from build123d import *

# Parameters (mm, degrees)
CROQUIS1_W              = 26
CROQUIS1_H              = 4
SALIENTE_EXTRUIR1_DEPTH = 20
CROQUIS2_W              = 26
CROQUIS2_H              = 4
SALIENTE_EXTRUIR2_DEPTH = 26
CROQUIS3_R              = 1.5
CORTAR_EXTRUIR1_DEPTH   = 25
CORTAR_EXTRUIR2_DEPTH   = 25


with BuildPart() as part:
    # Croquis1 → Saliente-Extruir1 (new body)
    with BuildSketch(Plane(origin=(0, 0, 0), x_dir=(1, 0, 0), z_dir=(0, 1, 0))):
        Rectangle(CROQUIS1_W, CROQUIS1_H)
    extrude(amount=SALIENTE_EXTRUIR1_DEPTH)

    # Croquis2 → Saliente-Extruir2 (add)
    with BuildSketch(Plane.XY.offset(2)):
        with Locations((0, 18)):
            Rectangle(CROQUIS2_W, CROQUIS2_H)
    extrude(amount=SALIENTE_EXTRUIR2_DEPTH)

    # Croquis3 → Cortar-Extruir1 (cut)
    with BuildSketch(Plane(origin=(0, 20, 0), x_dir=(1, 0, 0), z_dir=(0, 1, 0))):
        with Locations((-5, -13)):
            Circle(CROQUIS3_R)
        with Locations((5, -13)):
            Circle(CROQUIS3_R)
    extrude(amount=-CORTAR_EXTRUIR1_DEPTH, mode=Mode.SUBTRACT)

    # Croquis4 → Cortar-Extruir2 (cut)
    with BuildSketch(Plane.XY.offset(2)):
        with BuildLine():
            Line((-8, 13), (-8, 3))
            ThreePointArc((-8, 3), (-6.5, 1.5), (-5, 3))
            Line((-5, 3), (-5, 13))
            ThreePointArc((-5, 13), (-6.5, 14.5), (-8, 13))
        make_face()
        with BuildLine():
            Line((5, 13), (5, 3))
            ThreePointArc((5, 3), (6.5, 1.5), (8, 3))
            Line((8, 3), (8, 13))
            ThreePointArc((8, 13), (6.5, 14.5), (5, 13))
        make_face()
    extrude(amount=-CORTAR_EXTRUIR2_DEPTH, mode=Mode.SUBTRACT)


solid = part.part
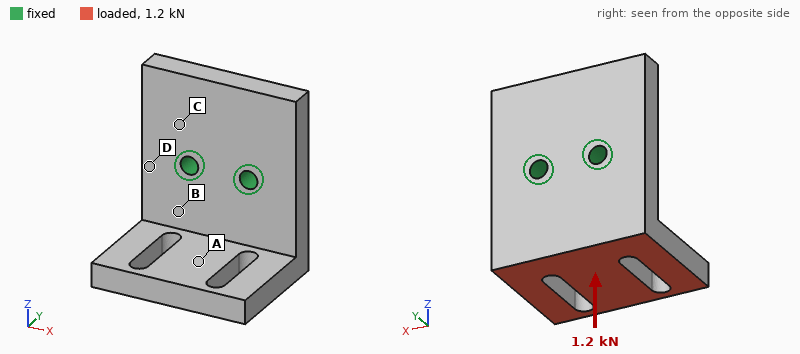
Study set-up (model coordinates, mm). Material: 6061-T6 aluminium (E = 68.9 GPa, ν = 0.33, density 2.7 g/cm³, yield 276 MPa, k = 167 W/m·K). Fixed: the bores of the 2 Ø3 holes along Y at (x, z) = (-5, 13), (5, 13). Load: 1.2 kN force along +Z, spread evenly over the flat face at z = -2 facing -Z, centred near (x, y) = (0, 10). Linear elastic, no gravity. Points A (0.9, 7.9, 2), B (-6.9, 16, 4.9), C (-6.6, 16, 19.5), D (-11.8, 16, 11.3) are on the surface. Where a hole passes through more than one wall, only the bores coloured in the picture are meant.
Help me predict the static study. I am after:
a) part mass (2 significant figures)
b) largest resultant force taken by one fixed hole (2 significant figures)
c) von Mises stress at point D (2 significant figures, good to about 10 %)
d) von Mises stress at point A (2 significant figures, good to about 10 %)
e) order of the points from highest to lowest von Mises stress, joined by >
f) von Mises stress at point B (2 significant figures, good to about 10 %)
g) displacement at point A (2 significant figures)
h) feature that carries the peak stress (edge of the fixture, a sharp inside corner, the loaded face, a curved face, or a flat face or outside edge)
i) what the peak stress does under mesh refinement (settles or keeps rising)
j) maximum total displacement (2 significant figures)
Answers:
12 g
610 N
86 MPa
36 MPa
B > D > A > C
130 MPa
0.16 mm
edge of the fixture
keeps rising
0.31 mm
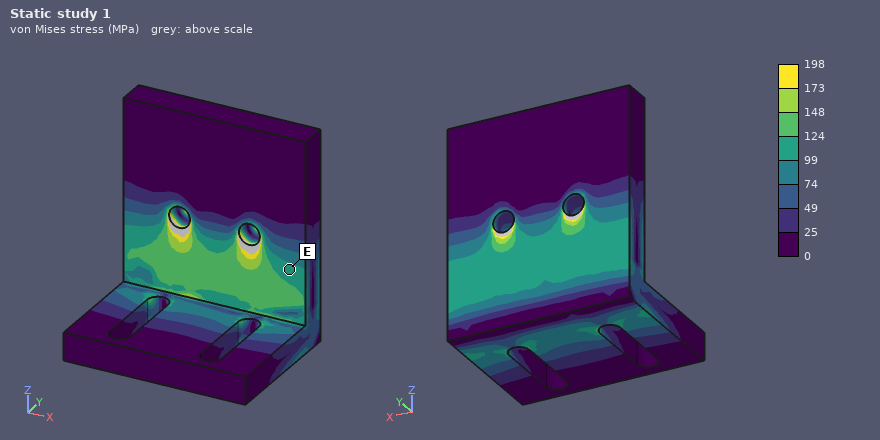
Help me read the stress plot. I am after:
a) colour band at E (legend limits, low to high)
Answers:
99 to 124 MPa
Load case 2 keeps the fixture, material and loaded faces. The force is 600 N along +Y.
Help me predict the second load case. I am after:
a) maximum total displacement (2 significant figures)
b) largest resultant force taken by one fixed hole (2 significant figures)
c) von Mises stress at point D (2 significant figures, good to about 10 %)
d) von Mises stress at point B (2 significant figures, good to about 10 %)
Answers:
0.15 mm
300 N
61 MPa
53 MPa
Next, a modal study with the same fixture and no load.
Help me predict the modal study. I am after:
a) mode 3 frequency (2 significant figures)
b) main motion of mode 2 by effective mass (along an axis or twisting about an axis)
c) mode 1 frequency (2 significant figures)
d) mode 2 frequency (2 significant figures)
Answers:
12 kHz
along X
4900 Hz
7500 Hz
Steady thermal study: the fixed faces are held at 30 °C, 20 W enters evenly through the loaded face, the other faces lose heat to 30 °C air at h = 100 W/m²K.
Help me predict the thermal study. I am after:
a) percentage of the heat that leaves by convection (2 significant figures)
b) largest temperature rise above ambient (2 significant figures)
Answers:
11 %
22 K
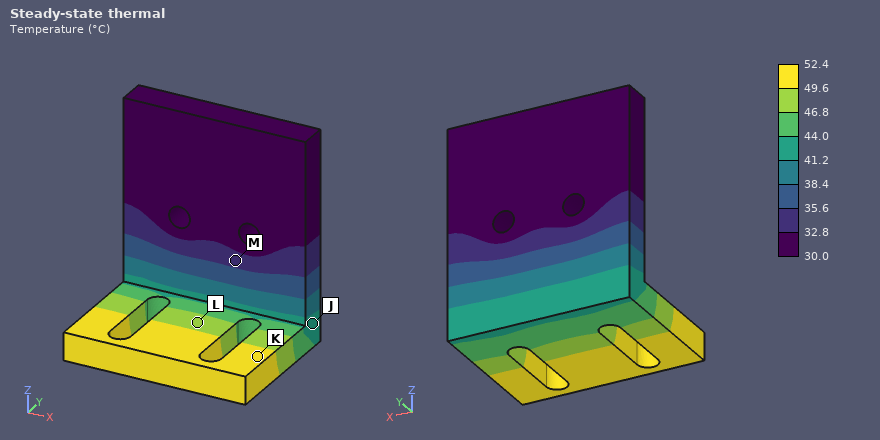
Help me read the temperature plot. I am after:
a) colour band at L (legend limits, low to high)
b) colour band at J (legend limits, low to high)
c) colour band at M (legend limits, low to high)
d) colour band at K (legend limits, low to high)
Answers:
46.8 to 49.6 °C
41.2 to 44.0 °C
32.8 to 35.6 °C
49.6 to 52.4 °C
